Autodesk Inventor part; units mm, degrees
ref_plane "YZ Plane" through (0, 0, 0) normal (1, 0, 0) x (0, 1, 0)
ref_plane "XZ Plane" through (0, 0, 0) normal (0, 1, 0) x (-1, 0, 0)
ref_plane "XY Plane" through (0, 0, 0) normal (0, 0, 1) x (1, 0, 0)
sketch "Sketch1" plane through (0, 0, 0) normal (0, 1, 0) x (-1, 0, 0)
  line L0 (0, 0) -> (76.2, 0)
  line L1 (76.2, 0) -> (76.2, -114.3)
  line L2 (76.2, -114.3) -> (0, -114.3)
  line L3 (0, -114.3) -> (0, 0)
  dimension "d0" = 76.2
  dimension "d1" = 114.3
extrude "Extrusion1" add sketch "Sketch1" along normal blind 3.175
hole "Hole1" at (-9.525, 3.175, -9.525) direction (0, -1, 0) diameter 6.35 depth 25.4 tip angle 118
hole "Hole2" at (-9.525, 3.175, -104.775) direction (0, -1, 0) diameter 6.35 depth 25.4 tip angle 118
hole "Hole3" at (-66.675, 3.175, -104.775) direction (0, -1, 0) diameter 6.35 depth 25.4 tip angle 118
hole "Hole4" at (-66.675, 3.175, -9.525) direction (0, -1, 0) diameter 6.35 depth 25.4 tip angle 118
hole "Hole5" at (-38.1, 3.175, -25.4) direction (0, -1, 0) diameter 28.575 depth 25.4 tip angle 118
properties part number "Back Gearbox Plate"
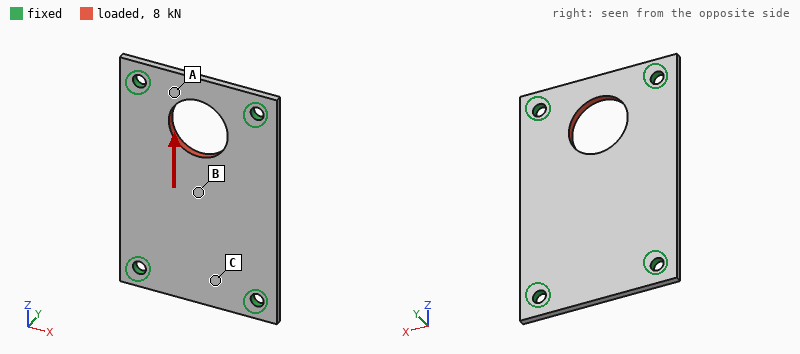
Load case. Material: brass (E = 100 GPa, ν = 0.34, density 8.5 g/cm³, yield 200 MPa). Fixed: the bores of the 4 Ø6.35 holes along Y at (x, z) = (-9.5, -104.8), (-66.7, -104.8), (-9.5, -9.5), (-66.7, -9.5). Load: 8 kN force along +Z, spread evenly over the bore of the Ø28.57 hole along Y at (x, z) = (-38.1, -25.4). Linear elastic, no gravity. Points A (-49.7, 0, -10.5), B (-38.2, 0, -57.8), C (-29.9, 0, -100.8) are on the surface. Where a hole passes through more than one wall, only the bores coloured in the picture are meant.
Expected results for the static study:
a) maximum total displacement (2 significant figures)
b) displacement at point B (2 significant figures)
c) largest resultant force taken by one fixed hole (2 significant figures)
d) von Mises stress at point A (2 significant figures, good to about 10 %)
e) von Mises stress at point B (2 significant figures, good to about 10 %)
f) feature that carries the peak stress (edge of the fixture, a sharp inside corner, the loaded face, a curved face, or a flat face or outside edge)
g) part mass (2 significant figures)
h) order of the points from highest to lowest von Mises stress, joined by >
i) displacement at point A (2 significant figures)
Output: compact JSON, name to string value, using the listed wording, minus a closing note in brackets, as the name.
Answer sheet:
{"maximum total displacement": "30 µm", "displacement at point B": "7.5 µm", "largest resultant force taken by one fixed hole": "2.8 kN", "von Mises stress at point A": "42 MPa", "von Mises stress at point B": "19 MPa", "feature that carries the peak stress": "edge of the fixture", "part mass": "210 g", "order of the points from highest to lowest von Mises stress, joined by >": "A > B > C", "displacement at point A": "19 µm"}
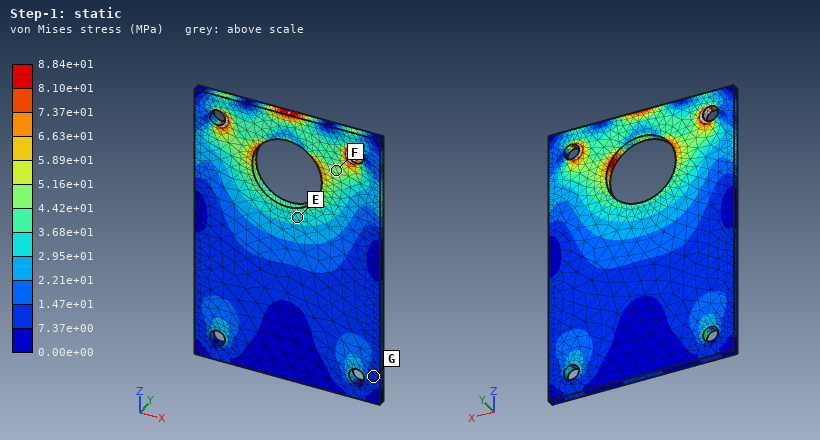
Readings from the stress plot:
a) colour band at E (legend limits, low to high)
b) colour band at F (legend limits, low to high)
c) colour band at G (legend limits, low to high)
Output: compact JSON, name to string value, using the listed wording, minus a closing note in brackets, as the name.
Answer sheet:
{"colour band at E": "2.95e+01 to 3.68e+01 MPa", "colour band at F": "4.42e+01 to 5.16e+01 MPa", "colour band at G": "7.37e+00 to 1.47e+01 MPa"}
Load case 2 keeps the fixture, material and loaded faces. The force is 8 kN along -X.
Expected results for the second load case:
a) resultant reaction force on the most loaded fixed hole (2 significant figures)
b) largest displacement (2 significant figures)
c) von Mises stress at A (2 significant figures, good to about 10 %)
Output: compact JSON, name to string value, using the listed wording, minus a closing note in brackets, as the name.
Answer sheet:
{"resultant reaction force on the most loaded fixed hole": "3.1 kN", "largest displacement": "26 µm", "von Mises stress at A": "40 MPa"}
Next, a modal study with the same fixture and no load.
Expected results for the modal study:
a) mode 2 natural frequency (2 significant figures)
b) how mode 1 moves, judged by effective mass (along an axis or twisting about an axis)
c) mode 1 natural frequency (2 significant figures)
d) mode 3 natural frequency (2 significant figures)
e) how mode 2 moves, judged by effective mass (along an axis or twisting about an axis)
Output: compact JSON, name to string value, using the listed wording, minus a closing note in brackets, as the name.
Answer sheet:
{"mode 2 natural frequency": "1600 Hz", "how mode 1 moves, judged by effective mass": "along Y", "mode 1 natural frequency": "1200 Hz", "mode 3 natural frequency": "2800 Hz", "how mode 2 moves, judged by effective mass": "twisting about Z"}
